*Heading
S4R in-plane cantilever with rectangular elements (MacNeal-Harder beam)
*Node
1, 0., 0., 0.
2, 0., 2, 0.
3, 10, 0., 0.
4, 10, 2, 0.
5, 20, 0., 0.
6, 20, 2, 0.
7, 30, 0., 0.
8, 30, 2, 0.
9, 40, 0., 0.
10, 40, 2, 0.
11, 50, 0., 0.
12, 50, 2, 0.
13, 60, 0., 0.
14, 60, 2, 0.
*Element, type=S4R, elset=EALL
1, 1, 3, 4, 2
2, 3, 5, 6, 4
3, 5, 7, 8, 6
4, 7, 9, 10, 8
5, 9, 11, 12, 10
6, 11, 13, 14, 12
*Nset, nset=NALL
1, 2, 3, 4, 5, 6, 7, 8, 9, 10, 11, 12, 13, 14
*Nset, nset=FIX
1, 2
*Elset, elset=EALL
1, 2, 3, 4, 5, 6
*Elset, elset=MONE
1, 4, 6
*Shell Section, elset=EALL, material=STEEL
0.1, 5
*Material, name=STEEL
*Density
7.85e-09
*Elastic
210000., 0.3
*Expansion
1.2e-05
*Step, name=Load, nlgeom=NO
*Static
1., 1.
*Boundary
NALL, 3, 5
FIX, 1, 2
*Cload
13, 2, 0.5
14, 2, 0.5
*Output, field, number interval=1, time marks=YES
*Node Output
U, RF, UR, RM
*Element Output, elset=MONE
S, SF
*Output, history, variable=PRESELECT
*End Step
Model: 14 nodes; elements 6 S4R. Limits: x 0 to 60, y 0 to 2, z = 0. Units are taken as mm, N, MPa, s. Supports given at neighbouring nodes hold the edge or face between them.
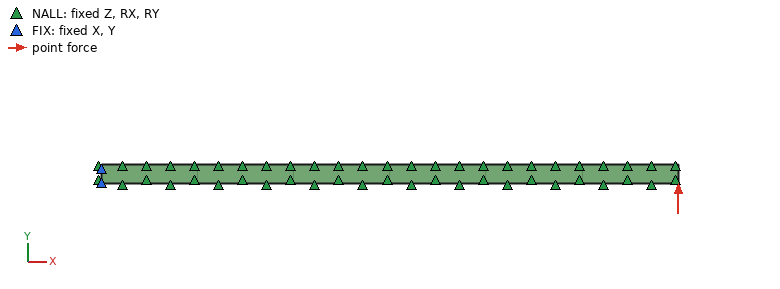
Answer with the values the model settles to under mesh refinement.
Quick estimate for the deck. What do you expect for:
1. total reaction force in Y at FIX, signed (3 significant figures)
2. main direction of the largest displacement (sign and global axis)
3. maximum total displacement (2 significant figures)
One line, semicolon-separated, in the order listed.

-1.00 N; +Y; 5.1 mm
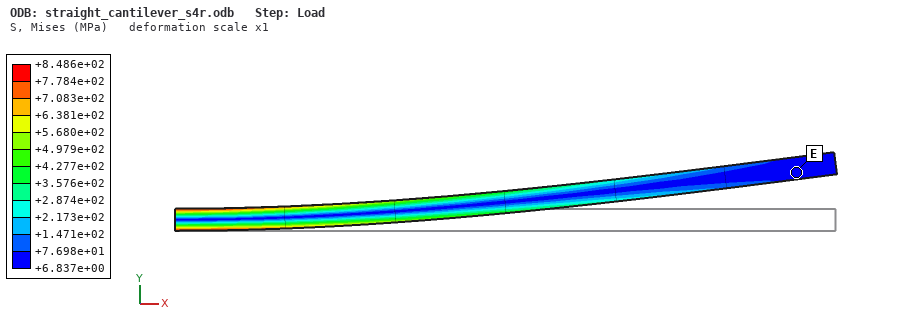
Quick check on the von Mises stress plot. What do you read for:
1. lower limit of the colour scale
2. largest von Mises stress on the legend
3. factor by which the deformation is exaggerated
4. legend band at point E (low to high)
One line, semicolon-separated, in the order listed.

+6.837e+00 MPa; +8.486e+02 MPa; 1; +6.837e+00 to +7.698e+01 MPa
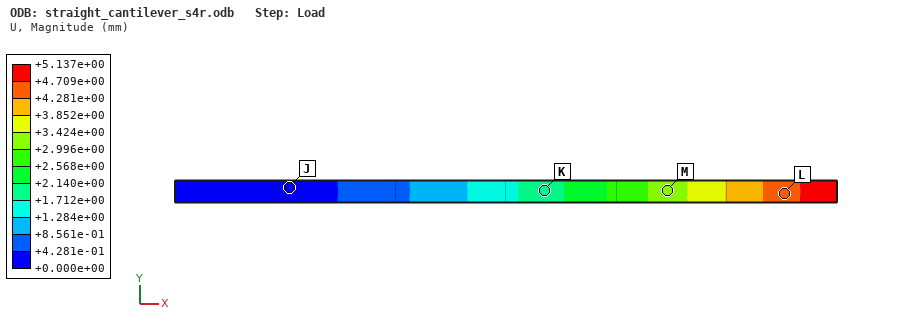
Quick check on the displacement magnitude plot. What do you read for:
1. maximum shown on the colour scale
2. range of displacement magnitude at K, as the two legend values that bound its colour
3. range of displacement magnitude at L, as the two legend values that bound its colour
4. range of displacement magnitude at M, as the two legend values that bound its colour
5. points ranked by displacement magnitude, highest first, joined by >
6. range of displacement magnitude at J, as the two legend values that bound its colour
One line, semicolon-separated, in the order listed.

+5.137e+00 mm; +1.712e+00 to +2.140e+00 mm; +4.281e+00 to +4.709e+00 mm; +2.996e+00 to +3.424e+00 mm; L > M > K > J; +0.000e+00 to +4.281e-01 mm
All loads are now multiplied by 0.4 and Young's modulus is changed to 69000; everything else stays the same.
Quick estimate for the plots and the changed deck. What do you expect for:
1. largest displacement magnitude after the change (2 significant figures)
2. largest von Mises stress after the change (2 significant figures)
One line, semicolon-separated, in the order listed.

6.3 mm; 340 MPa
